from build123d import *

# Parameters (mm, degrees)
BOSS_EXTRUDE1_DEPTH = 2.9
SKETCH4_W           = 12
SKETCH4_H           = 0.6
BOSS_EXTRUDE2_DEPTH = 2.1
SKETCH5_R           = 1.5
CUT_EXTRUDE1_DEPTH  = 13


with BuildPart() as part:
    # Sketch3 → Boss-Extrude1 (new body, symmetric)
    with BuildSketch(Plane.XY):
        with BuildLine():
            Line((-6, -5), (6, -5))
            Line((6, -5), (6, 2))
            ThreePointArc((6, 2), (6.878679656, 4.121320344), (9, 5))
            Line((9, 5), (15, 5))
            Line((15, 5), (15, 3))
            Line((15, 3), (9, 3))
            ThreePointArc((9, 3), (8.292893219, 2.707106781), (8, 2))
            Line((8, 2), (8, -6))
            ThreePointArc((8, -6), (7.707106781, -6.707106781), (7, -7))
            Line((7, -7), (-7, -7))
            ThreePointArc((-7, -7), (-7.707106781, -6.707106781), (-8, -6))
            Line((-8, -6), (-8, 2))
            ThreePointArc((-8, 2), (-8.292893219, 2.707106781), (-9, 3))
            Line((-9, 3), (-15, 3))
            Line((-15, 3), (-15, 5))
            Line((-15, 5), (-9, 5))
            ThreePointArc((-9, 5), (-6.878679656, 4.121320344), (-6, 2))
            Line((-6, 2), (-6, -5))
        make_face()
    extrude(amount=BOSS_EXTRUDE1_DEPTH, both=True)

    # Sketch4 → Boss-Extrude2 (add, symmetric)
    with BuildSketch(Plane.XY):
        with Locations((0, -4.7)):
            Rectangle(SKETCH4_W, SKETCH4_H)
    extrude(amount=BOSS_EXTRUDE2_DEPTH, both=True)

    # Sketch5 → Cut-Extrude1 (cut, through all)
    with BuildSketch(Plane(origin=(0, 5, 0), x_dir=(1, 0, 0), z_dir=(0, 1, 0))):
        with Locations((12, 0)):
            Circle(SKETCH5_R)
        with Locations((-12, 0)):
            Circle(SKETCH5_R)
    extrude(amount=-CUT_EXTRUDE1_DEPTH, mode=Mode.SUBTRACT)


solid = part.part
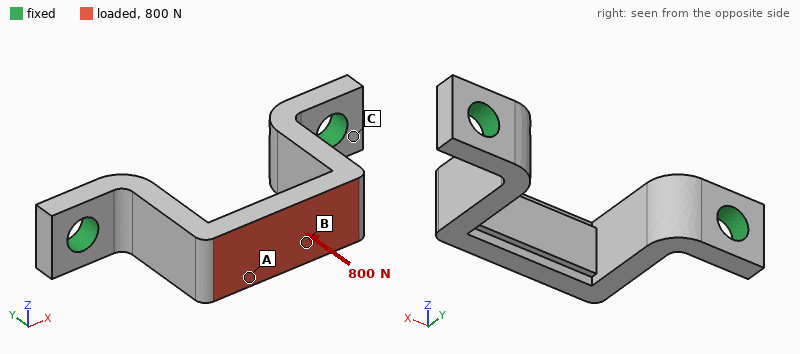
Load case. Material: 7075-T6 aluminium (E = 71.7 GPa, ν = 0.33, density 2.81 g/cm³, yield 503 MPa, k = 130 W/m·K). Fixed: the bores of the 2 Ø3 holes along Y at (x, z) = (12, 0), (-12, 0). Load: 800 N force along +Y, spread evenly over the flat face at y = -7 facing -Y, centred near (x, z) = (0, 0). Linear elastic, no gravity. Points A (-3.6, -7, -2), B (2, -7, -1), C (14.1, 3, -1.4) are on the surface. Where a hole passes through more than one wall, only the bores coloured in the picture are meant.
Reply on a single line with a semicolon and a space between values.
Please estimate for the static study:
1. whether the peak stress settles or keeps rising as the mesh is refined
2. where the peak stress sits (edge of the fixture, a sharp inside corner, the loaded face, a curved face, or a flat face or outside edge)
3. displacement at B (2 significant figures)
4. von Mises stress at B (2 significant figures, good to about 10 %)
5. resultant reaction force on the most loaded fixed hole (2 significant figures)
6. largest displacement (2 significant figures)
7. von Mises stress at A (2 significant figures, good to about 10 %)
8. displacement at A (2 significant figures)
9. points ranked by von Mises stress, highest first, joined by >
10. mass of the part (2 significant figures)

keeps rising; edge of the fixture; 37 µm; 99 MPa; 430 N; 42 µm; 58 MPa; 33 µm; B > A > C; 1.6 g
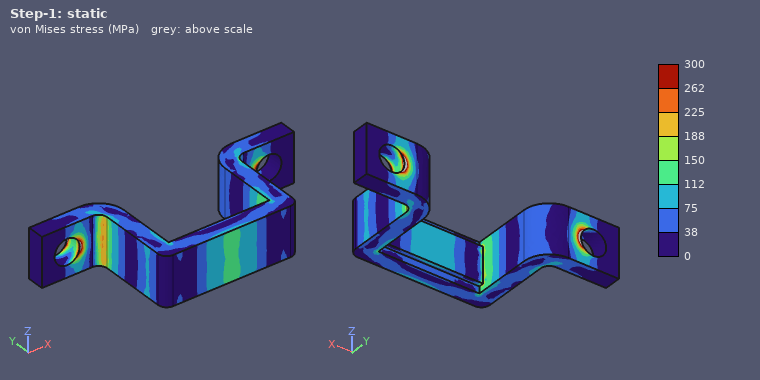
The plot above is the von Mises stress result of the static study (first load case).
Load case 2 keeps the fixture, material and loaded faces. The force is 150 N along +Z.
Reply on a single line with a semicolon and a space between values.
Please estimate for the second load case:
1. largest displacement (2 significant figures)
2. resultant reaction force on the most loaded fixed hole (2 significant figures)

91 µm; 75 N
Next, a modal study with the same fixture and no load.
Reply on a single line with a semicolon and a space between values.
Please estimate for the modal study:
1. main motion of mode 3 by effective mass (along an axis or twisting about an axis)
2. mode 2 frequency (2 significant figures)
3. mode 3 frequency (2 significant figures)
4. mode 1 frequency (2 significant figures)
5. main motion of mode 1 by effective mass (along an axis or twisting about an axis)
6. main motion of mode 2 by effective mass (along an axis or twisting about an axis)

twisting about Y; 12 kHz; 17 kHz; 8400 Hz; along Z; along X
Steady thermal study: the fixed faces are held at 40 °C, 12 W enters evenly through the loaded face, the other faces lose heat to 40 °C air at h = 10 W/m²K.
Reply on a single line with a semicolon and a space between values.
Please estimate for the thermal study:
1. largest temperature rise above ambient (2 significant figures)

59 K
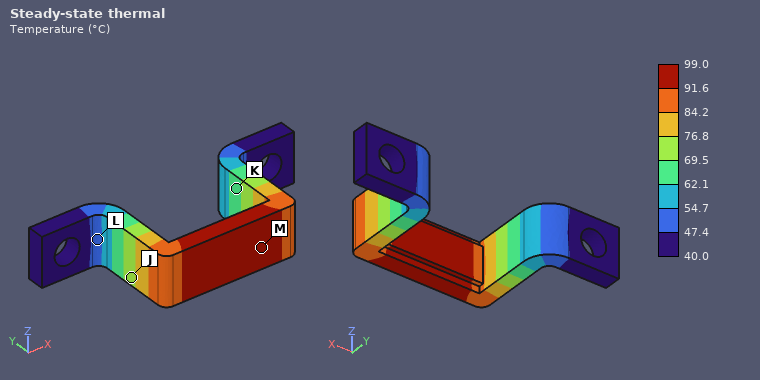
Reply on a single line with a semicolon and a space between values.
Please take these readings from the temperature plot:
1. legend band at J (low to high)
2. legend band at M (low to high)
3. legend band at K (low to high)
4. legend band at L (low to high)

69.5 to 76.8 °C; 91.6 to 99.0 °C; 62.1 to 69.5 °C; 47.4 to 54.7 °C
